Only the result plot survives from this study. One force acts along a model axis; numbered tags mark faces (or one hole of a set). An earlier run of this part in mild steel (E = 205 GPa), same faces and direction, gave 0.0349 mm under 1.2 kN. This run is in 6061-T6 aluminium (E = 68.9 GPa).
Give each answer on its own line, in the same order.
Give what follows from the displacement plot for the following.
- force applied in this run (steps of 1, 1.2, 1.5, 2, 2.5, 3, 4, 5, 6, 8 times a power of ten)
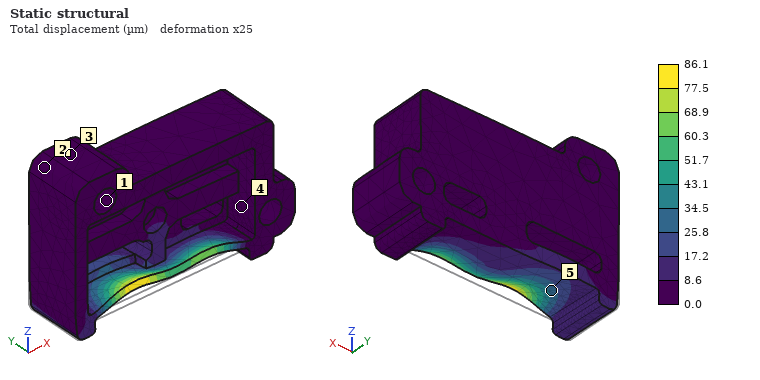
1 kN
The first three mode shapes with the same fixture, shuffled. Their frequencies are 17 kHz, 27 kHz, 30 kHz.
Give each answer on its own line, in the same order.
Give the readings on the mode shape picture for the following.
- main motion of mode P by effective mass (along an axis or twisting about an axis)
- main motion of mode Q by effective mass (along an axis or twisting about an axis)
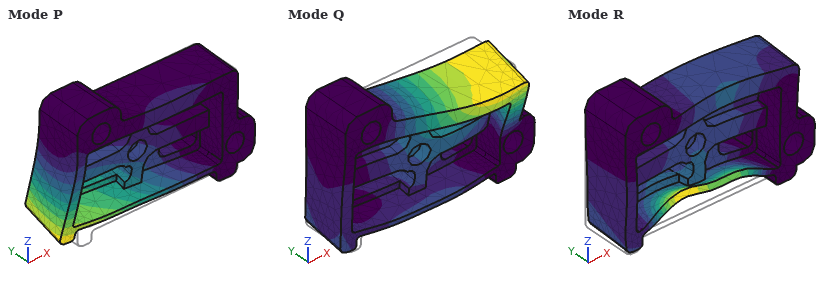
along Y
along Y
